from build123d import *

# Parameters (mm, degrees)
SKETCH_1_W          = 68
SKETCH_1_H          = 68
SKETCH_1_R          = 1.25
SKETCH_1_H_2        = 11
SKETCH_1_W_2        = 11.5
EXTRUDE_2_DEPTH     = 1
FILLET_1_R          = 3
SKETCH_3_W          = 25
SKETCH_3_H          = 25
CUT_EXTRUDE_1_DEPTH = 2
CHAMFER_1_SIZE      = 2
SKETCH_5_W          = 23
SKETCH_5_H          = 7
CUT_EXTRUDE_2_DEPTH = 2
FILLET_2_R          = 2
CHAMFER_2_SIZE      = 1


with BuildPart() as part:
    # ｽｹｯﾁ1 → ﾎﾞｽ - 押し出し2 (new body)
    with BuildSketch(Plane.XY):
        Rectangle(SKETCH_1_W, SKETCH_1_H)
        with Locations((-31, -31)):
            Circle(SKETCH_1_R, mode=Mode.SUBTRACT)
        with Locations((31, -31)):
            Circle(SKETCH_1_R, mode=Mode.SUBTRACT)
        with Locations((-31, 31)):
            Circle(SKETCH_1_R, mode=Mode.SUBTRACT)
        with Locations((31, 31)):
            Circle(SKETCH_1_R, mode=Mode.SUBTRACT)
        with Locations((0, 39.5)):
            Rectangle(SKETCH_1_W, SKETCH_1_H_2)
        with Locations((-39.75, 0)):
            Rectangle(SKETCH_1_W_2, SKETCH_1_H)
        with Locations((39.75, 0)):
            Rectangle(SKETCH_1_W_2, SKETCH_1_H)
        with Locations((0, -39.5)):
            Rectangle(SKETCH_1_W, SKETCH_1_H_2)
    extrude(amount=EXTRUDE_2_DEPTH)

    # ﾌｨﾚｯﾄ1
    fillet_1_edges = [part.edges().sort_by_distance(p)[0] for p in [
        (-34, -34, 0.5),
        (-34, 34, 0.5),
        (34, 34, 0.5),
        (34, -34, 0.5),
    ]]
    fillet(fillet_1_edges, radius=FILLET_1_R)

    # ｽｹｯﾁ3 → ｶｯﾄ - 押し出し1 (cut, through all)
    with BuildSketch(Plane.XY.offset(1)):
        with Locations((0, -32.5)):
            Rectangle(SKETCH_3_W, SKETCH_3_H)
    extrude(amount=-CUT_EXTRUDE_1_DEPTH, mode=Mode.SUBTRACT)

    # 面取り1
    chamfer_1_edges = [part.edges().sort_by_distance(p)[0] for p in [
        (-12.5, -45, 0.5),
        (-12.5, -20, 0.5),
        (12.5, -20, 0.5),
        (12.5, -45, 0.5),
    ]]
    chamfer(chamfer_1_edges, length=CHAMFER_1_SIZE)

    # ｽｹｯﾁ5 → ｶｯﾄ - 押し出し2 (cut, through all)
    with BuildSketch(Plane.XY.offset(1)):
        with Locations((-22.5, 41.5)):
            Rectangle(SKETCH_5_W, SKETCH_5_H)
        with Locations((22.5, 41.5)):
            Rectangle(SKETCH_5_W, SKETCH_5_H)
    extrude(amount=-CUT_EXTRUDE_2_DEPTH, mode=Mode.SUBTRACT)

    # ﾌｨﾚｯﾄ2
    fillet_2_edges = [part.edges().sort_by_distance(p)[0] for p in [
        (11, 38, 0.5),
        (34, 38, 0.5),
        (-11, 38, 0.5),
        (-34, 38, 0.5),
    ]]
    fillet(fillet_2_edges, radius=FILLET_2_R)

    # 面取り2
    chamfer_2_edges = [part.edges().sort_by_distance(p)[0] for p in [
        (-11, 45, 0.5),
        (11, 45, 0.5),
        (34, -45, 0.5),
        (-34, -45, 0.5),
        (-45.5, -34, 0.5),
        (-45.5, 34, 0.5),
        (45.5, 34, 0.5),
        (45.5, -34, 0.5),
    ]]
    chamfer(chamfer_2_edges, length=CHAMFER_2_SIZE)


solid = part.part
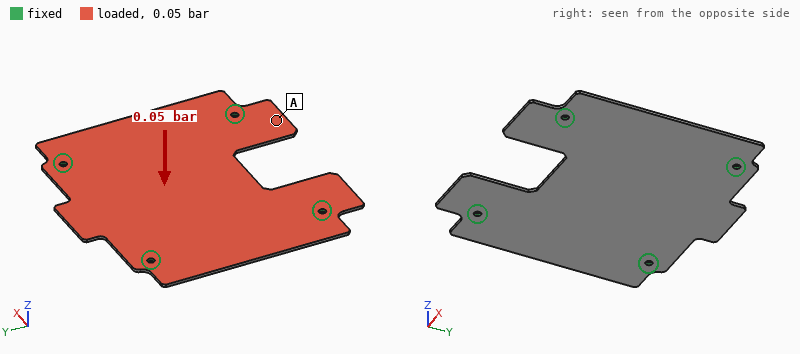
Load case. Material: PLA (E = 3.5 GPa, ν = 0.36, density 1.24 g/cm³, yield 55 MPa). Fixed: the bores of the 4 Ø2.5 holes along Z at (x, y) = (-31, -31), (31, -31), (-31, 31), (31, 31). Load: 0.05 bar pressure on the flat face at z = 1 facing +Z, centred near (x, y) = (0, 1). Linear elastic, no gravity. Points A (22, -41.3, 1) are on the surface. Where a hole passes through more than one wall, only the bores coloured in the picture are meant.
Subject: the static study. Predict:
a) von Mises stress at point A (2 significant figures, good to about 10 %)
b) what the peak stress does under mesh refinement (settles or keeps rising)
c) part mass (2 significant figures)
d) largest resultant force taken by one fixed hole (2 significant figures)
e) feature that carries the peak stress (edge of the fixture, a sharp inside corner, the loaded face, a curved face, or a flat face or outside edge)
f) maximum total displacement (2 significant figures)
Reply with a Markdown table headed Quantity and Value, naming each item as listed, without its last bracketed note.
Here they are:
| Quantity | Value |
|---|---|
| von Mises stress at point A | 2.7 MPa |
| what the peak stress does under mesh refinement | keeps rising |
| part mass | 8.3 g |
| largest resultant force taken by one fixed hole | 8.7 N |
| feature that carries the peak stress | edge of the fixture |
| maximum total displacement | 1.5 mm |
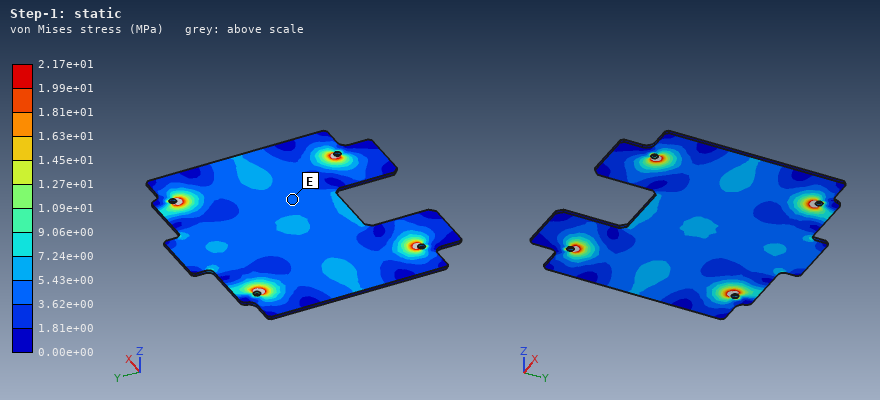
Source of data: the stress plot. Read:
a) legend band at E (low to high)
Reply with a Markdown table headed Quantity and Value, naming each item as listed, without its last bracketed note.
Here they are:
| Quantity | Value |
|---|---|
| legend band at E | 3.62e+00 to 5.43e+00 MPa |
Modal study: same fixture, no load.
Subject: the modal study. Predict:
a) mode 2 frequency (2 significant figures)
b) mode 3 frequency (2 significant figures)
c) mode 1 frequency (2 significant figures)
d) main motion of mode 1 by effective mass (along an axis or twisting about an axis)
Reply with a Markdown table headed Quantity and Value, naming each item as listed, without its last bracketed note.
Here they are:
| Quantity | Value |
|---|---|
| mode 2 frequency | 420 Hz |
| mode 3 frequency | 430 Hz |
| mode 1 frequency | 310 Hz |
| main motion of mode 1 by effective mass | along Z |
